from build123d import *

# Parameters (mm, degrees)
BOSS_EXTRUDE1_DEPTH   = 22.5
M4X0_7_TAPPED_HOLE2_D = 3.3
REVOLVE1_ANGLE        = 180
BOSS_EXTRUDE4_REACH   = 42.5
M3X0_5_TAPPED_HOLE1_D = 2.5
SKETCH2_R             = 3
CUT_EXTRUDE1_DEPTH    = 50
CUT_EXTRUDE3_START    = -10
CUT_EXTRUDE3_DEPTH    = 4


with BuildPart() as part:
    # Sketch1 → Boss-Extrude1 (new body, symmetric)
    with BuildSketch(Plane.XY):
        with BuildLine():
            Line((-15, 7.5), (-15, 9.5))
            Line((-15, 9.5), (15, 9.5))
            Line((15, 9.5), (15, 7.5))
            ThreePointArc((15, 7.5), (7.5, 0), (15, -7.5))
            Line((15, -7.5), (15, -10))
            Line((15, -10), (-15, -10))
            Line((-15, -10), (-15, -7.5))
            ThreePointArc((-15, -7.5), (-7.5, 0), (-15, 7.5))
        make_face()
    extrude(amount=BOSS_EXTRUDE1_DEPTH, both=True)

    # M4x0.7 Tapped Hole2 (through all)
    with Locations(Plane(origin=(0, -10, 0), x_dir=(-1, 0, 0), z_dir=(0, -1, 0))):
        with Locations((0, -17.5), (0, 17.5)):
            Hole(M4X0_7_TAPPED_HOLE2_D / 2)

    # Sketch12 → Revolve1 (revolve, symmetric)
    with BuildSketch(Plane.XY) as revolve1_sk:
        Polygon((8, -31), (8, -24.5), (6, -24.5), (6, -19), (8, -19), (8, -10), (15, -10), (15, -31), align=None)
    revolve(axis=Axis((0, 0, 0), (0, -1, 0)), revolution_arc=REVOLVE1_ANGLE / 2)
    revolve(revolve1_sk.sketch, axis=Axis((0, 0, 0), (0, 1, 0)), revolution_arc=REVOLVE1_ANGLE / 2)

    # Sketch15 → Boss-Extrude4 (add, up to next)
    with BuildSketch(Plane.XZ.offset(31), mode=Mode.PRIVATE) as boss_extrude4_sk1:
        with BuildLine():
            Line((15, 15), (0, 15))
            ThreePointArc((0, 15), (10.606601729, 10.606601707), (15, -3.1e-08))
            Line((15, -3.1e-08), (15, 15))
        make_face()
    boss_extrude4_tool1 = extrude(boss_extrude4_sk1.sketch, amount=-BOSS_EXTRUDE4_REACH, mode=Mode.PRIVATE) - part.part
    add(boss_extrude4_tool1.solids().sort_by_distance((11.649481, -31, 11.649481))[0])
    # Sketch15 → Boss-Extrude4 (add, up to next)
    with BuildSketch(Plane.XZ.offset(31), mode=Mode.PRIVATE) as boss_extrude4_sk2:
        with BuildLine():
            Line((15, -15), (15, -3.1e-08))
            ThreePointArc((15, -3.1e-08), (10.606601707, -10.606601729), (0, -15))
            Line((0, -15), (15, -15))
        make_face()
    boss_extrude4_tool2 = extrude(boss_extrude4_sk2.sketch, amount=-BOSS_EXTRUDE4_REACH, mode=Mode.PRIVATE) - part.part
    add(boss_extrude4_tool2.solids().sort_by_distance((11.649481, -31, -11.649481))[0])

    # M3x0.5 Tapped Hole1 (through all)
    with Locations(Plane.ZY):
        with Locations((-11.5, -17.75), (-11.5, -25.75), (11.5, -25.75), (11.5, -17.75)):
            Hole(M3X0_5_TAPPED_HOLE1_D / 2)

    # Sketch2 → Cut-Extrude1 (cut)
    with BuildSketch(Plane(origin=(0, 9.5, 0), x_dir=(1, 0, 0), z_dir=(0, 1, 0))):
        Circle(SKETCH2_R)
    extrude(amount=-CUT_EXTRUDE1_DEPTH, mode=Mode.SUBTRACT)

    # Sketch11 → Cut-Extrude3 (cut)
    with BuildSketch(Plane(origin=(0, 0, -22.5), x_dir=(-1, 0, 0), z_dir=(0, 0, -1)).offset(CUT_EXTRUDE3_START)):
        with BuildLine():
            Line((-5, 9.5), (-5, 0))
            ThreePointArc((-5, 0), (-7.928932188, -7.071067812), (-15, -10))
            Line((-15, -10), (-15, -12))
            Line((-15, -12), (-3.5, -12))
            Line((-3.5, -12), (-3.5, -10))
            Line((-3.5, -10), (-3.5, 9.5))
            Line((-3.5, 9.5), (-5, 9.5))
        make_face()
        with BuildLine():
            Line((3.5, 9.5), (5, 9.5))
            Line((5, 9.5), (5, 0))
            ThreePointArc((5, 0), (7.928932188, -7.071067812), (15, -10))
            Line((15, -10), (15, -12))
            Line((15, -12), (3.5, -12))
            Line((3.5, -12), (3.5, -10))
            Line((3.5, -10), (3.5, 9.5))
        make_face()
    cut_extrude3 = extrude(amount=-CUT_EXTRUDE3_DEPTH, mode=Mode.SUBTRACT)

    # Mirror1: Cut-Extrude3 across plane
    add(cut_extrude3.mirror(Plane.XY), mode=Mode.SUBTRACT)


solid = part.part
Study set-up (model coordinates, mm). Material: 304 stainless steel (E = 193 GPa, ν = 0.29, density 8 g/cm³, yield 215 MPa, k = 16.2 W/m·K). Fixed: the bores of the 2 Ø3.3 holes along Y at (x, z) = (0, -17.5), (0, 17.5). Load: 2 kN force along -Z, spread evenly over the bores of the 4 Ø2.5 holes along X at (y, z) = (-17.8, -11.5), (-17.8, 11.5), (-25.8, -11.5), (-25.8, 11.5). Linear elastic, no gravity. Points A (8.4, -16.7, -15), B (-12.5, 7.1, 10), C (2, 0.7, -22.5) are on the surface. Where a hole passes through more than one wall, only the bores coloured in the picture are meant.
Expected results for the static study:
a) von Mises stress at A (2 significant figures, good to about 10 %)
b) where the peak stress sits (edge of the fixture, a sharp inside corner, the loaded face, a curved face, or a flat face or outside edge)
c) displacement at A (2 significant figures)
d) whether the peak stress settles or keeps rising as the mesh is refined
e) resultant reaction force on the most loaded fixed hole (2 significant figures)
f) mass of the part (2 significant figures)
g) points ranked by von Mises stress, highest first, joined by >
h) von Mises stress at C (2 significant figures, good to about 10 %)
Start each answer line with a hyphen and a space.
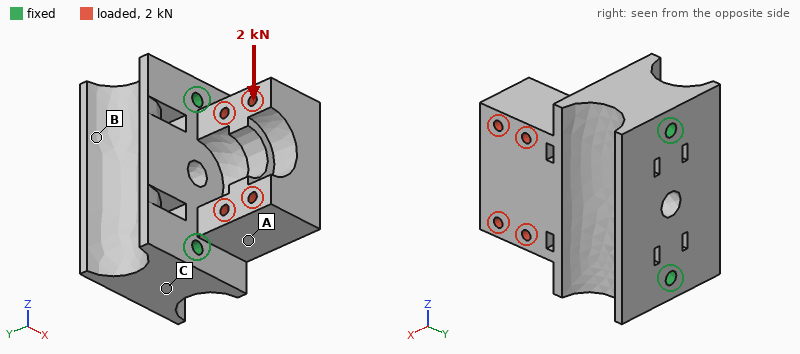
- 11 MPa
- a sharp inside corner
- 3.5 µm
- keeps rising
- 1.5 kN
- 190 g
- A > C > B
- 8.6 MPa
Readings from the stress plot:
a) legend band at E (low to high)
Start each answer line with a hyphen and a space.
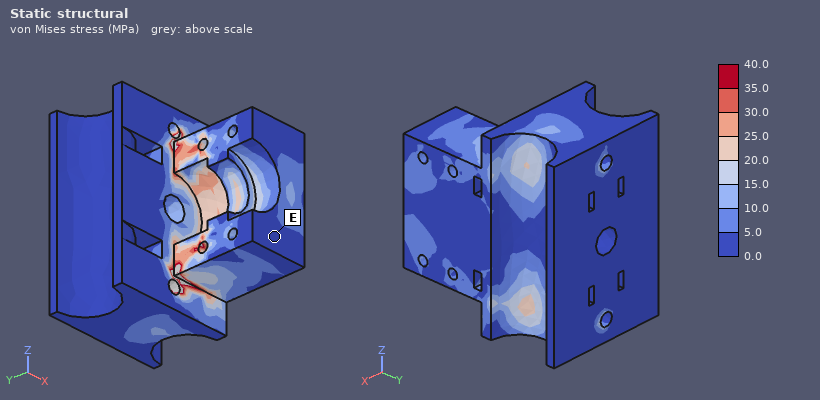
- 0.0 to 5.0 MPa
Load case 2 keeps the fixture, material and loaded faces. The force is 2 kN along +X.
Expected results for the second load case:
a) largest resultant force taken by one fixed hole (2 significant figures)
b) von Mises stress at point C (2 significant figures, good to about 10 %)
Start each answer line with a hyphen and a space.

- 1.0 kN
- 11 MPa
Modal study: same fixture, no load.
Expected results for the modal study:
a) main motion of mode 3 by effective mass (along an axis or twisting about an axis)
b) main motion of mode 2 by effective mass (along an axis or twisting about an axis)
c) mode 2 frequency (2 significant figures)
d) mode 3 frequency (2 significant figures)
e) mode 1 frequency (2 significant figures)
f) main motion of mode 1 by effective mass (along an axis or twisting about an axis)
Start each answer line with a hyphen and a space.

- along Z
- along Z
- 14 kHz
- 20 kHz
- 7900 Hz
- along X
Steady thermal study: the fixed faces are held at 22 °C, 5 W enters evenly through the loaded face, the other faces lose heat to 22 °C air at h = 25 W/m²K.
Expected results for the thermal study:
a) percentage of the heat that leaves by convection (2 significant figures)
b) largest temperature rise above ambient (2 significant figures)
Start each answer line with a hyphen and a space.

- 27 %
- 19 K
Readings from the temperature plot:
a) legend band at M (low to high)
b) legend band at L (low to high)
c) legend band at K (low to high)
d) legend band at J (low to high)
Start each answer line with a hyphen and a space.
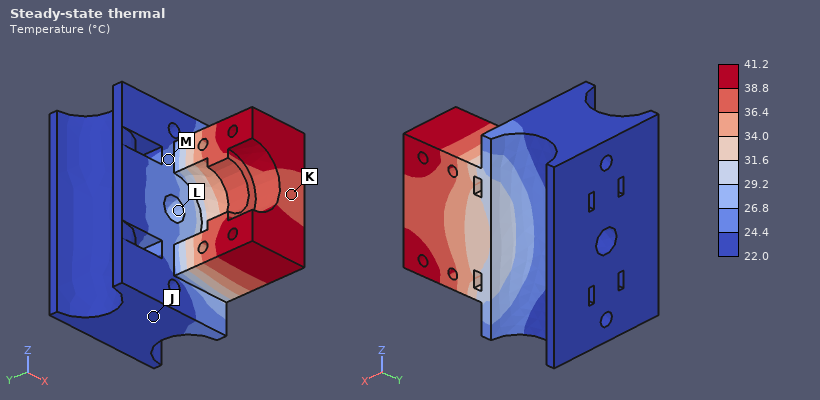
- 24.4 to 26.8 °C
- 26.8 to 29.2 °C
- 36.4 to 38.8 °C
- 22.0 to 24.4 °C
